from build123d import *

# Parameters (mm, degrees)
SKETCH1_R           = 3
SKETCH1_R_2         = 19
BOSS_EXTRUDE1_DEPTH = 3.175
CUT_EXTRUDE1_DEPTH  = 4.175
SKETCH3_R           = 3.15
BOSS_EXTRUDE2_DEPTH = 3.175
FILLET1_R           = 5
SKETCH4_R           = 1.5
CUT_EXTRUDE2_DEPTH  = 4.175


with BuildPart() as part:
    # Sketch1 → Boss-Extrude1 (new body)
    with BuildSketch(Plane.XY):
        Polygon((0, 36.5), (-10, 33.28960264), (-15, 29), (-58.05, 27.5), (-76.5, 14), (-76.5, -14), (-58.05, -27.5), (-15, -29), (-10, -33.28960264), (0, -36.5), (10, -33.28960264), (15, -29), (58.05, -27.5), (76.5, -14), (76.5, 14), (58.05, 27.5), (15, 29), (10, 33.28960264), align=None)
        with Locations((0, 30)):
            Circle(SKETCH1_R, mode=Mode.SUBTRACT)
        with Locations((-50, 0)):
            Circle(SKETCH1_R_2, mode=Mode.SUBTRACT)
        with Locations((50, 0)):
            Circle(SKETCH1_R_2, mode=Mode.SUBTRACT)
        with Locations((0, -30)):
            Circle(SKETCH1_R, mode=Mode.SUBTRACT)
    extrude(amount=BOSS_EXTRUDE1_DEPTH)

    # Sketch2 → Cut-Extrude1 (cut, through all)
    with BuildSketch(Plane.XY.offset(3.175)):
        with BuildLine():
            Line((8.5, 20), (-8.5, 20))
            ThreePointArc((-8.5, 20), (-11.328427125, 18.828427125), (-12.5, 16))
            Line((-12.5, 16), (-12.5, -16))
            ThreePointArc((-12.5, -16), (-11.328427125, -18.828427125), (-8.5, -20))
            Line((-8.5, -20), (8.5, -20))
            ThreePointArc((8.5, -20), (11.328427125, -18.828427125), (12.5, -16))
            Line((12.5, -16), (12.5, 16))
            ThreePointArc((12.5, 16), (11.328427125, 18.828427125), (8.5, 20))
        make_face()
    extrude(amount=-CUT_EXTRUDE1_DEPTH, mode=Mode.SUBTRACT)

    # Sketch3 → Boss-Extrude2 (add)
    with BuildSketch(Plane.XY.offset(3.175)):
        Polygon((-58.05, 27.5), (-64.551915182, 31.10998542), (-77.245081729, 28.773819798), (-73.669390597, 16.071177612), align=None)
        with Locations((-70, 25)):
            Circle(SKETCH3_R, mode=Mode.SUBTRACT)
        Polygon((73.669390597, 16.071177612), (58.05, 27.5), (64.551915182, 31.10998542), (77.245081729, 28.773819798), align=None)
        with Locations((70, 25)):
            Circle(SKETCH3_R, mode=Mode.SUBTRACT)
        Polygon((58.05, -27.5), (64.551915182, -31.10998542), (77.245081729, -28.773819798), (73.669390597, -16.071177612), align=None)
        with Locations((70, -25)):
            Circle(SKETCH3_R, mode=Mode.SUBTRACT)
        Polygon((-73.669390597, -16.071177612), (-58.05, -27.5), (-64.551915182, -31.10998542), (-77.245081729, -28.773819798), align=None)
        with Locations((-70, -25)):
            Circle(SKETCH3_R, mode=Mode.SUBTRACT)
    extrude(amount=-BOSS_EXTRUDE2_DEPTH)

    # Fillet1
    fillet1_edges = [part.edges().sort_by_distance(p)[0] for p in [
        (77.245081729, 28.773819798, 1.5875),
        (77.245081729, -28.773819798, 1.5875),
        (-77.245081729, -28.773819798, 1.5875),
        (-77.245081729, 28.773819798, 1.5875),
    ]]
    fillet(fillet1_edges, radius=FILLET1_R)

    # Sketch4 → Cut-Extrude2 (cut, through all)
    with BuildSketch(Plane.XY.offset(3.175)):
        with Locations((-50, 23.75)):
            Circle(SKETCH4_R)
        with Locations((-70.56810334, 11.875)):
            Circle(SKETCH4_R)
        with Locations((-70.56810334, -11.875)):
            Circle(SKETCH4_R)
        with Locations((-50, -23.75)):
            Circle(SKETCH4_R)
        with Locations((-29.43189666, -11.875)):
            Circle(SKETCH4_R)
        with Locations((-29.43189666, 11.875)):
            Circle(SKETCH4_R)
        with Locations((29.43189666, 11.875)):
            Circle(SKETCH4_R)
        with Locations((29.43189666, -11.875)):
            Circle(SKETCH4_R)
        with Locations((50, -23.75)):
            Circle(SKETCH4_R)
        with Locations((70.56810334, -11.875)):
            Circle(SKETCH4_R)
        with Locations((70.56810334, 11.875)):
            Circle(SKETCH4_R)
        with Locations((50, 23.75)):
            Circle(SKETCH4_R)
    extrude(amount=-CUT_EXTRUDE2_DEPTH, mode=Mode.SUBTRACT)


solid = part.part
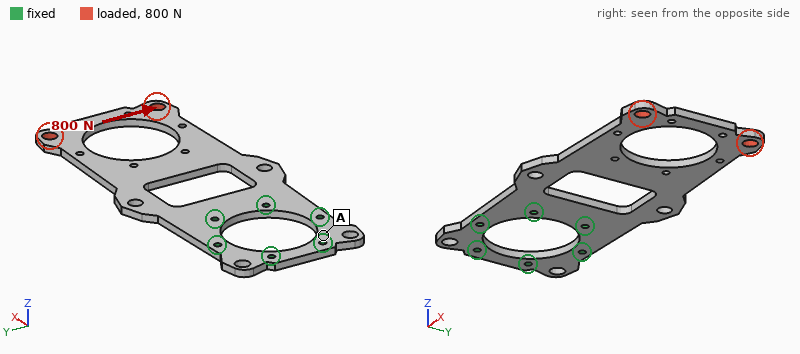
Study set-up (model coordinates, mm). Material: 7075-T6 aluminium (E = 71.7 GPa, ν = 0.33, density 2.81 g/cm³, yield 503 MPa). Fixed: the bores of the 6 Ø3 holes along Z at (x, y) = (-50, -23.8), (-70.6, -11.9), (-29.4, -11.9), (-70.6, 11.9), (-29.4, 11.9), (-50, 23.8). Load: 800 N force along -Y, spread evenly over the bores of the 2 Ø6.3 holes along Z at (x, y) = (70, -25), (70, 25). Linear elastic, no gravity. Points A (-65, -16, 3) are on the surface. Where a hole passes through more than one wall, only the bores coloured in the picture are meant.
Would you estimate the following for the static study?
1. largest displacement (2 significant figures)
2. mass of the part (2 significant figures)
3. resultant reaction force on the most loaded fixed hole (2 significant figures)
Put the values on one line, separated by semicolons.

0.37 mm; 49 g; 1.1 kN
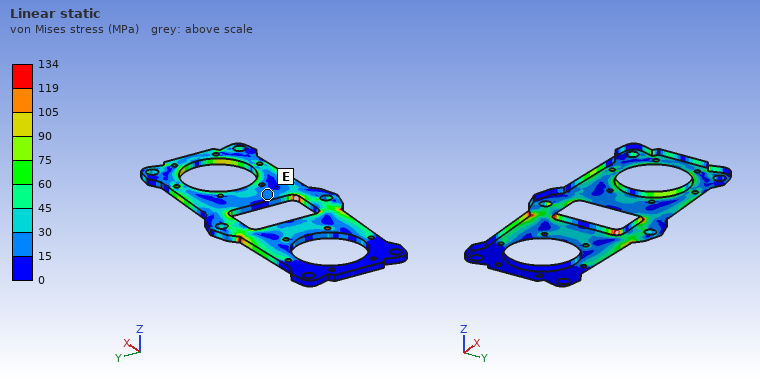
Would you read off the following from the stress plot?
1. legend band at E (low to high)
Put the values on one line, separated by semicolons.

15 to 30 MPa
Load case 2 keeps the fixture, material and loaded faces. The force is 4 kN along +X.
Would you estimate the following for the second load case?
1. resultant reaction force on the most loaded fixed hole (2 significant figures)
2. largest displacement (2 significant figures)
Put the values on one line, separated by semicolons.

1.2 kN; 0.11 mm
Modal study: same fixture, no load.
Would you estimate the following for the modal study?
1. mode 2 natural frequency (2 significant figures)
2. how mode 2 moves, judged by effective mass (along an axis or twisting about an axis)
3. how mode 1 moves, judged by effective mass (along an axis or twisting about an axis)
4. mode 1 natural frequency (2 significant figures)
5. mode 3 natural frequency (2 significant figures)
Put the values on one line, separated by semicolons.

740 Hz; twisting about X; along Z; 210 Hz; 1200 Hz
